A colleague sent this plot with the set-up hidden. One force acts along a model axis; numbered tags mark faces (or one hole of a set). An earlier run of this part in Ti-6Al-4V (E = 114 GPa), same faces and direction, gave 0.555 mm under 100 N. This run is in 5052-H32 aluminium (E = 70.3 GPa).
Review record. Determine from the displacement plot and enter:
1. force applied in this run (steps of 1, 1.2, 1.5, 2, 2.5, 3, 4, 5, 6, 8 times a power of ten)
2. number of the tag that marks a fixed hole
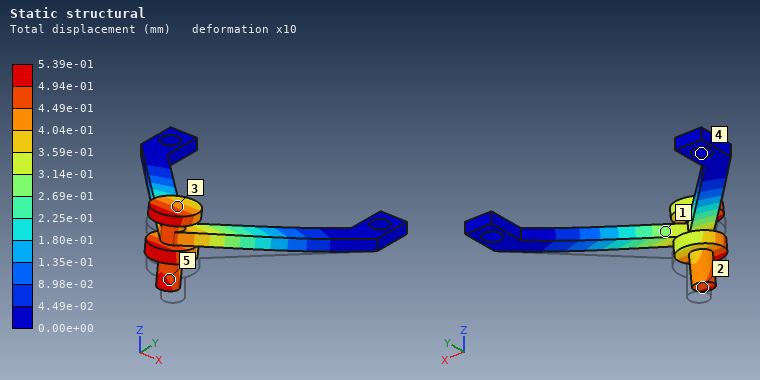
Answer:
60 N
4
